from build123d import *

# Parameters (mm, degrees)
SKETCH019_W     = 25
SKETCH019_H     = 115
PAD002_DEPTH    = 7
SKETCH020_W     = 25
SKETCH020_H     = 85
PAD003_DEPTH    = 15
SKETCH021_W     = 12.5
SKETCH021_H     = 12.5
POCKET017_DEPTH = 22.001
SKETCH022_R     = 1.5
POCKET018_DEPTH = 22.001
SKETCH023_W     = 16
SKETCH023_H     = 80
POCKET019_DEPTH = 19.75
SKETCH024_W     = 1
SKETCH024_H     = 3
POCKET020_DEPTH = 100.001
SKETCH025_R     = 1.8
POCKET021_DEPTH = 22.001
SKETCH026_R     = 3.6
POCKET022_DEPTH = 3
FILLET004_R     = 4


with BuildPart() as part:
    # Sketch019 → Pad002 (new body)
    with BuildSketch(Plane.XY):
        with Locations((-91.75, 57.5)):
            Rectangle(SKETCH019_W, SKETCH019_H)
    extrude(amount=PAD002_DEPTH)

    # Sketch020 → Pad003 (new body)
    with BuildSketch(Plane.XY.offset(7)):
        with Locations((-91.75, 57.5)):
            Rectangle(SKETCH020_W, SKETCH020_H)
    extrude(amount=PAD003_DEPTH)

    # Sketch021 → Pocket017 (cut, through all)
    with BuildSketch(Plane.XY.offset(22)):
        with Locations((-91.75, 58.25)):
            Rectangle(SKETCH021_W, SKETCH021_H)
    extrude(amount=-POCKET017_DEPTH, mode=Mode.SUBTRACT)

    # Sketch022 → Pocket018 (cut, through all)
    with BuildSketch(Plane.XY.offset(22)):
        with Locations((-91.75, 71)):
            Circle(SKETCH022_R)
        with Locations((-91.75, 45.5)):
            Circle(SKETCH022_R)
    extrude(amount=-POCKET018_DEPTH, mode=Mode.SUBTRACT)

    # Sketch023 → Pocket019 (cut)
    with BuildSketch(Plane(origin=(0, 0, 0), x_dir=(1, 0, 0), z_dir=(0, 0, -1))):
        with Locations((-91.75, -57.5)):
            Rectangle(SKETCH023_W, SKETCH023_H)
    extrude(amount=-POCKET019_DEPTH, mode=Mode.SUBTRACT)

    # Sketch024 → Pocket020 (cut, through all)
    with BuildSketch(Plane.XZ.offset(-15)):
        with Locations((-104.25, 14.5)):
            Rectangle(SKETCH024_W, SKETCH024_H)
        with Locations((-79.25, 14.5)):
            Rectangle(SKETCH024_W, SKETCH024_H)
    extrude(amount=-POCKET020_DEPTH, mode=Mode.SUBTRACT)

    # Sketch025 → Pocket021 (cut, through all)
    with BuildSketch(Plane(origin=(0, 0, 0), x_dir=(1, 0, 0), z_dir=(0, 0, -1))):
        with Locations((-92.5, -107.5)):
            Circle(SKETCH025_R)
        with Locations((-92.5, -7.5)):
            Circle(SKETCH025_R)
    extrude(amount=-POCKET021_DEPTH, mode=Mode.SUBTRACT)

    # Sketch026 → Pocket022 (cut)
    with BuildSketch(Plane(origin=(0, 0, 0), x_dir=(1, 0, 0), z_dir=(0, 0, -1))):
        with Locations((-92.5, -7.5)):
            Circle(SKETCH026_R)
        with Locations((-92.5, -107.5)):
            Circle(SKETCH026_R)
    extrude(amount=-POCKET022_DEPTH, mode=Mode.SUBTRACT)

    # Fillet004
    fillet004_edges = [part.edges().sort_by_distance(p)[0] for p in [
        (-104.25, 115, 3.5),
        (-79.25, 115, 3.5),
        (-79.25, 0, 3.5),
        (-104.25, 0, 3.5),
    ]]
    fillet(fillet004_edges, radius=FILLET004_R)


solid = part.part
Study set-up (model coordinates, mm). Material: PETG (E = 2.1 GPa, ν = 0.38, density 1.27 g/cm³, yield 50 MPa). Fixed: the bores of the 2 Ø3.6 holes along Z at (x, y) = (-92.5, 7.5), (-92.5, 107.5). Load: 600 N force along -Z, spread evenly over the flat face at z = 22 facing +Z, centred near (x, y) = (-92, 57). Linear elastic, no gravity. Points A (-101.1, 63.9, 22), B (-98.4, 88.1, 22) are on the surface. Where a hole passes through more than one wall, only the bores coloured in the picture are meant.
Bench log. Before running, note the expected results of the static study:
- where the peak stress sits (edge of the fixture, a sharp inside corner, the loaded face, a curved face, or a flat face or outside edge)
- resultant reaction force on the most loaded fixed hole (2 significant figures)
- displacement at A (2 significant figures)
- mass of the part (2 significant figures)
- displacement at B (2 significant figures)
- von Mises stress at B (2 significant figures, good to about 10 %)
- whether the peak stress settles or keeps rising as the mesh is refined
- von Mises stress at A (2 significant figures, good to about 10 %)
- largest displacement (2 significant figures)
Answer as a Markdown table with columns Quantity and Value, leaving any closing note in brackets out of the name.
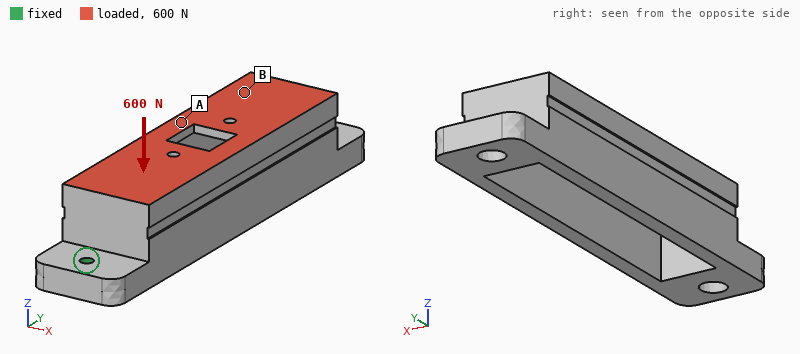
| Quantity | Value |
|---|---|
| where the peak stress sits | edge of the fixture |
| resultant reaction force on the most loaded fixed hole | 360 N |
| displacement at A | 0.39 mm |
| mass of the part | 33 g |
| displacement at B | 0.30 mm |
| von Mises stress at B | 2.8 MPa |
| whether the peak stress settles or keeps rising as the mesh is refined | keeps rising |
| von Mises stress at A | 7.4 MPa |
| largest displacement | 0.52 mm |
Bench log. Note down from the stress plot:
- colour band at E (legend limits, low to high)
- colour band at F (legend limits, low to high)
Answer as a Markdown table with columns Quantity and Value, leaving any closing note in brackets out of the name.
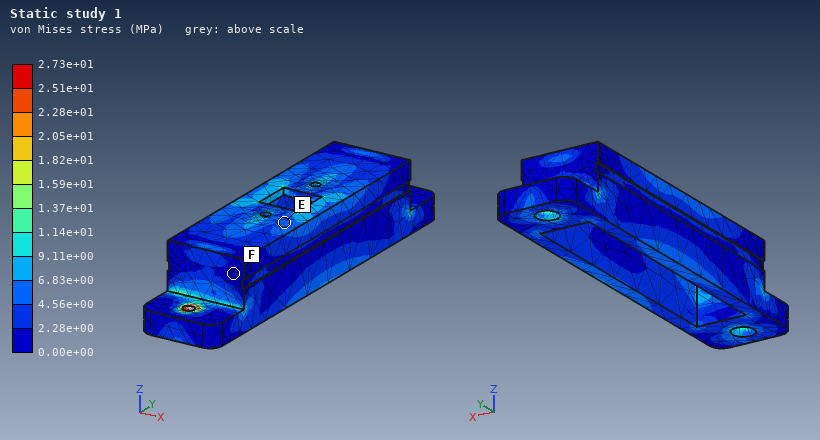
| Quantity | Value |
|---|---|
| colour band at E | 4.56e+00 to 6.83e+00 MPa |
| colour band at F | 0.00e+00 to 2.28e+00 MPa |
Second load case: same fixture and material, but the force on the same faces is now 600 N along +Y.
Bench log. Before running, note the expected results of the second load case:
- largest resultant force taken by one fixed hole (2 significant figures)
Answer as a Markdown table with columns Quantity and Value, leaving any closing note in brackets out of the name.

| Quantity | Value |
|---|---|
| largest resultant force taken by one fixed hole | 320 N |
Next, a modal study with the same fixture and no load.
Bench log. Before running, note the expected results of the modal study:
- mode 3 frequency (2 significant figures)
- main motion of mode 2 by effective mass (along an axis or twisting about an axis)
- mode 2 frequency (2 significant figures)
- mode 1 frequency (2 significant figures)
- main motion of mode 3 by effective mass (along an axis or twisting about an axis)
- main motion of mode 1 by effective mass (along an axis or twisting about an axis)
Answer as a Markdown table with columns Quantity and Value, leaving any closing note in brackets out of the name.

| Quantity | Value |
|---|---|
| mode 3 frequency | 1300 Hz |
| main motion of mode 2 by effective mass | along X |
| mode 2 frequency | 1200 Hz |
| mode 1 frequency | 800 Hz |
| main motion of mode 3 by effective mass | along Z |
| main motion of mode 1 by effective mass | along X |
